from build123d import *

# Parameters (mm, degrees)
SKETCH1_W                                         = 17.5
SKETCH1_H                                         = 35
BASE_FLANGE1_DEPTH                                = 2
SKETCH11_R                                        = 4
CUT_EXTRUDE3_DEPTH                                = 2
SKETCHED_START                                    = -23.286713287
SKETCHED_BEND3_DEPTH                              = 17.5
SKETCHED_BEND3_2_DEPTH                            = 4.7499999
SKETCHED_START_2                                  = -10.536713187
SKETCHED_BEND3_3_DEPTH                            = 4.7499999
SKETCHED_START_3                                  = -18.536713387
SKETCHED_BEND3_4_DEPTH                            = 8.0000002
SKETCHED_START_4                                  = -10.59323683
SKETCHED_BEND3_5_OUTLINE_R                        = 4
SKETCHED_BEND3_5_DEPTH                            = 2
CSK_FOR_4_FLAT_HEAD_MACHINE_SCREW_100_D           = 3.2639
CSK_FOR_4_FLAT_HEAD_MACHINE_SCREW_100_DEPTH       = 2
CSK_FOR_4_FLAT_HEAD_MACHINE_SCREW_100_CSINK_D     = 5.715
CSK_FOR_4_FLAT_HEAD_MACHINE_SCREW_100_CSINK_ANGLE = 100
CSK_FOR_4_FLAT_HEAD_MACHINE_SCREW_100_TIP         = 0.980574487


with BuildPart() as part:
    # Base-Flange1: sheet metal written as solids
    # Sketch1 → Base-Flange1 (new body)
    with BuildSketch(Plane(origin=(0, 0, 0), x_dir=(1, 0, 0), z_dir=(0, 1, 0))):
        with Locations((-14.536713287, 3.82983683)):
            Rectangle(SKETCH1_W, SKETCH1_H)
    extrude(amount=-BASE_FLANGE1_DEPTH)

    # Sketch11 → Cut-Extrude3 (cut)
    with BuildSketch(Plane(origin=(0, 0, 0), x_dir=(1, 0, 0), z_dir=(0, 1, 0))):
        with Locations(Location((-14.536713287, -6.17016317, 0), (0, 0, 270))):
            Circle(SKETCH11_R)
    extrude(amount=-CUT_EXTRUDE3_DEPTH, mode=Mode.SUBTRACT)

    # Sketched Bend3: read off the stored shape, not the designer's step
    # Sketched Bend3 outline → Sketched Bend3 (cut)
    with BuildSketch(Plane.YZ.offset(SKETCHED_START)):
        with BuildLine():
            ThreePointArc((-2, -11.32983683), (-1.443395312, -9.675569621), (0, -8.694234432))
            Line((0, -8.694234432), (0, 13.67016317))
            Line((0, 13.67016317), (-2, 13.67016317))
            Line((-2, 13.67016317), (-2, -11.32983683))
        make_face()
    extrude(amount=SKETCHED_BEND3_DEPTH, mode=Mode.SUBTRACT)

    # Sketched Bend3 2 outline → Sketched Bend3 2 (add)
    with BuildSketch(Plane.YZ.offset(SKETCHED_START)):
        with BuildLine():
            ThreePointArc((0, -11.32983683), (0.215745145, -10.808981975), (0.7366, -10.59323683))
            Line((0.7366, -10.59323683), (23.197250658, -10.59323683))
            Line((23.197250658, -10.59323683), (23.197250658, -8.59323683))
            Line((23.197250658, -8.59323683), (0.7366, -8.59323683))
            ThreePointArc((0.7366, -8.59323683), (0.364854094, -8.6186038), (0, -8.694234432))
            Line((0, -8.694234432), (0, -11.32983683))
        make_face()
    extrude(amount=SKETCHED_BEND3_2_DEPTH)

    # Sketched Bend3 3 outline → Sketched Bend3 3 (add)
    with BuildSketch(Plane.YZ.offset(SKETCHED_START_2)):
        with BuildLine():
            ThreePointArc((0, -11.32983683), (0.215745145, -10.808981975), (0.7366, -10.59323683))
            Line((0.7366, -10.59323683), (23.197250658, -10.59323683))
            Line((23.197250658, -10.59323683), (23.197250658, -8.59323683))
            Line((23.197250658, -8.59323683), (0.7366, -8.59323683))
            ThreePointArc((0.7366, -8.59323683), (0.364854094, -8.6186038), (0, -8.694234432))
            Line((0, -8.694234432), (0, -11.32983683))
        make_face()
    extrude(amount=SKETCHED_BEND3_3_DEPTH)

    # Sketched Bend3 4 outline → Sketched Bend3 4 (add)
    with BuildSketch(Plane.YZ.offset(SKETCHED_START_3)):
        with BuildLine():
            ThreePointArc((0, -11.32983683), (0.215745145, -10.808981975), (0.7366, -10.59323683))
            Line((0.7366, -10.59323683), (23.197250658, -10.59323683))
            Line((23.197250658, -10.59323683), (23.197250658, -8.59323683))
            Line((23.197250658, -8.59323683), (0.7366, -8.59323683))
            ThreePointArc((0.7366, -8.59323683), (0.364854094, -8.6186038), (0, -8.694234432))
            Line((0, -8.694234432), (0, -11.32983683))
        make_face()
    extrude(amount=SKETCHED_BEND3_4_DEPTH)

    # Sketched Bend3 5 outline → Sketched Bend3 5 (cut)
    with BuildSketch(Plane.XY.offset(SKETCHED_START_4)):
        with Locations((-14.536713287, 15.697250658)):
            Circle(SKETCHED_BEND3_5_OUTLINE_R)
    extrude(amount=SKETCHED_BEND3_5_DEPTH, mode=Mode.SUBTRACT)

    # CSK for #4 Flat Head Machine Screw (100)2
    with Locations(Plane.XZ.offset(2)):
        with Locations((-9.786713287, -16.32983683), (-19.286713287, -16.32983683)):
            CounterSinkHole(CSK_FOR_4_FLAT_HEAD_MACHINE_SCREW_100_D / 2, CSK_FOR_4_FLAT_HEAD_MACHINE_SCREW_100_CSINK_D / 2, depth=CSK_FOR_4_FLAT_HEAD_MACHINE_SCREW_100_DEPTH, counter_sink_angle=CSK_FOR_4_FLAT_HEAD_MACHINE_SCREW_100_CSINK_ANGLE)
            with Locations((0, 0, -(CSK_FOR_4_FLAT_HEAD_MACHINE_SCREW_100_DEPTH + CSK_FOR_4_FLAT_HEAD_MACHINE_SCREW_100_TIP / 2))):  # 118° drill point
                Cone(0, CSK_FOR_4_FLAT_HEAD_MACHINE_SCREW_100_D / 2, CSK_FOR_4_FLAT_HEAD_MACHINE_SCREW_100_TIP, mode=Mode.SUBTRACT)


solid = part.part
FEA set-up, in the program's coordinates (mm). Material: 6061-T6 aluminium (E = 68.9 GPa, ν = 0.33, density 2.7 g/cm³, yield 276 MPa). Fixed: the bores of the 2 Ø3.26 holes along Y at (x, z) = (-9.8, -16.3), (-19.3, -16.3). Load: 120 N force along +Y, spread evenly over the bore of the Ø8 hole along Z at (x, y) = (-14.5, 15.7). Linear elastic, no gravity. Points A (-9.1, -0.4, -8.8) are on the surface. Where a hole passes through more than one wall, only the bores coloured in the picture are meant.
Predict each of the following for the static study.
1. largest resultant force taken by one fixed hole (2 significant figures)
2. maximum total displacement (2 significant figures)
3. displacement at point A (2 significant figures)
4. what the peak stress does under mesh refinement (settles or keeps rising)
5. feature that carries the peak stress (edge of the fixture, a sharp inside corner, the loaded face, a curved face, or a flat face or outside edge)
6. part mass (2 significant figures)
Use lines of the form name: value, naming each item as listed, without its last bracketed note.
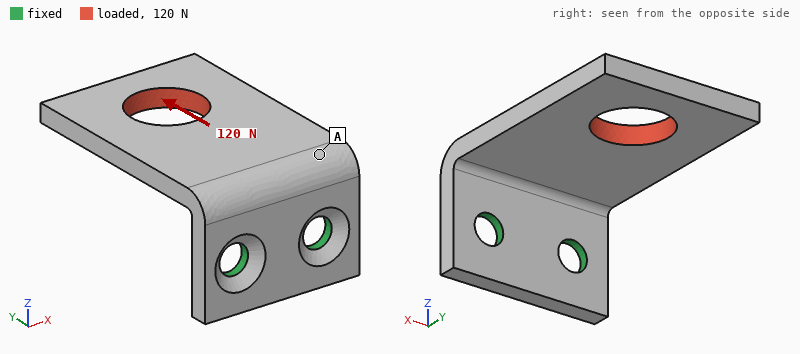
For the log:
largest resultant force taken by one fixed hole: 61 N
maximum total displacement: 0.10 mm
displacement at point A: 0.023 mm
what the peak stress does under mesh refinement: keeps rising
feature that carries the peak stress: edge of the fixture
part mass: 2.9 g
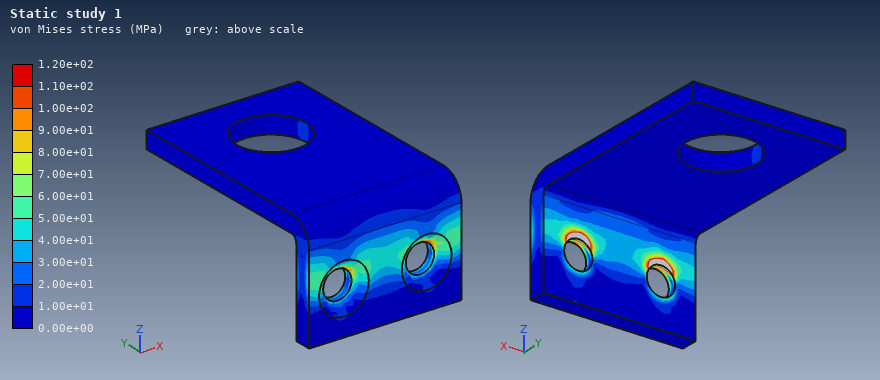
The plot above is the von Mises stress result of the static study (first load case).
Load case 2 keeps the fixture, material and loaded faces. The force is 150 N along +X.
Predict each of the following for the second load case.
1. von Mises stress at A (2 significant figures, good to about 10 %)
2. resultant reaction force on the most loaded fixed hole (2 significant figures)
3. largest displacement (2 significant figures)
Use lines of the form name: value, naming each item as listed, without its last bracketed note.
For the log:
von Mises stress at A: 57 MPa
resultant reaction force on the most loaded fixed hole: 230 N
largest displacement: 0.16 mm
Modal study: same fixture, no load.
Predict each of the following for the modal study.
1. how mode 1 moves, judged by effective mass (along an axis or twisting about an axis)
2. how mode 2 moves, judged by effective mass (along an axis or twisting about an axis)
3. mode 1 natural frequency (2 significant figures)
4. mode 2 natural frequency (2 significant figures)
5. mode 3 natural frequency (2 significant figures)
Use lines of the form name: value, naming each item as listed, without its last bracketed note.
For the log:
how mode 1 moves, judged by effective mass: along Z
how mode 2 moves, judged by effective mass: along X
mode 1 natural frequency: 2100 Hz
mode 2 natural frequency: 4900 Hz
mode 3 natural frequency: 7800 Hz
